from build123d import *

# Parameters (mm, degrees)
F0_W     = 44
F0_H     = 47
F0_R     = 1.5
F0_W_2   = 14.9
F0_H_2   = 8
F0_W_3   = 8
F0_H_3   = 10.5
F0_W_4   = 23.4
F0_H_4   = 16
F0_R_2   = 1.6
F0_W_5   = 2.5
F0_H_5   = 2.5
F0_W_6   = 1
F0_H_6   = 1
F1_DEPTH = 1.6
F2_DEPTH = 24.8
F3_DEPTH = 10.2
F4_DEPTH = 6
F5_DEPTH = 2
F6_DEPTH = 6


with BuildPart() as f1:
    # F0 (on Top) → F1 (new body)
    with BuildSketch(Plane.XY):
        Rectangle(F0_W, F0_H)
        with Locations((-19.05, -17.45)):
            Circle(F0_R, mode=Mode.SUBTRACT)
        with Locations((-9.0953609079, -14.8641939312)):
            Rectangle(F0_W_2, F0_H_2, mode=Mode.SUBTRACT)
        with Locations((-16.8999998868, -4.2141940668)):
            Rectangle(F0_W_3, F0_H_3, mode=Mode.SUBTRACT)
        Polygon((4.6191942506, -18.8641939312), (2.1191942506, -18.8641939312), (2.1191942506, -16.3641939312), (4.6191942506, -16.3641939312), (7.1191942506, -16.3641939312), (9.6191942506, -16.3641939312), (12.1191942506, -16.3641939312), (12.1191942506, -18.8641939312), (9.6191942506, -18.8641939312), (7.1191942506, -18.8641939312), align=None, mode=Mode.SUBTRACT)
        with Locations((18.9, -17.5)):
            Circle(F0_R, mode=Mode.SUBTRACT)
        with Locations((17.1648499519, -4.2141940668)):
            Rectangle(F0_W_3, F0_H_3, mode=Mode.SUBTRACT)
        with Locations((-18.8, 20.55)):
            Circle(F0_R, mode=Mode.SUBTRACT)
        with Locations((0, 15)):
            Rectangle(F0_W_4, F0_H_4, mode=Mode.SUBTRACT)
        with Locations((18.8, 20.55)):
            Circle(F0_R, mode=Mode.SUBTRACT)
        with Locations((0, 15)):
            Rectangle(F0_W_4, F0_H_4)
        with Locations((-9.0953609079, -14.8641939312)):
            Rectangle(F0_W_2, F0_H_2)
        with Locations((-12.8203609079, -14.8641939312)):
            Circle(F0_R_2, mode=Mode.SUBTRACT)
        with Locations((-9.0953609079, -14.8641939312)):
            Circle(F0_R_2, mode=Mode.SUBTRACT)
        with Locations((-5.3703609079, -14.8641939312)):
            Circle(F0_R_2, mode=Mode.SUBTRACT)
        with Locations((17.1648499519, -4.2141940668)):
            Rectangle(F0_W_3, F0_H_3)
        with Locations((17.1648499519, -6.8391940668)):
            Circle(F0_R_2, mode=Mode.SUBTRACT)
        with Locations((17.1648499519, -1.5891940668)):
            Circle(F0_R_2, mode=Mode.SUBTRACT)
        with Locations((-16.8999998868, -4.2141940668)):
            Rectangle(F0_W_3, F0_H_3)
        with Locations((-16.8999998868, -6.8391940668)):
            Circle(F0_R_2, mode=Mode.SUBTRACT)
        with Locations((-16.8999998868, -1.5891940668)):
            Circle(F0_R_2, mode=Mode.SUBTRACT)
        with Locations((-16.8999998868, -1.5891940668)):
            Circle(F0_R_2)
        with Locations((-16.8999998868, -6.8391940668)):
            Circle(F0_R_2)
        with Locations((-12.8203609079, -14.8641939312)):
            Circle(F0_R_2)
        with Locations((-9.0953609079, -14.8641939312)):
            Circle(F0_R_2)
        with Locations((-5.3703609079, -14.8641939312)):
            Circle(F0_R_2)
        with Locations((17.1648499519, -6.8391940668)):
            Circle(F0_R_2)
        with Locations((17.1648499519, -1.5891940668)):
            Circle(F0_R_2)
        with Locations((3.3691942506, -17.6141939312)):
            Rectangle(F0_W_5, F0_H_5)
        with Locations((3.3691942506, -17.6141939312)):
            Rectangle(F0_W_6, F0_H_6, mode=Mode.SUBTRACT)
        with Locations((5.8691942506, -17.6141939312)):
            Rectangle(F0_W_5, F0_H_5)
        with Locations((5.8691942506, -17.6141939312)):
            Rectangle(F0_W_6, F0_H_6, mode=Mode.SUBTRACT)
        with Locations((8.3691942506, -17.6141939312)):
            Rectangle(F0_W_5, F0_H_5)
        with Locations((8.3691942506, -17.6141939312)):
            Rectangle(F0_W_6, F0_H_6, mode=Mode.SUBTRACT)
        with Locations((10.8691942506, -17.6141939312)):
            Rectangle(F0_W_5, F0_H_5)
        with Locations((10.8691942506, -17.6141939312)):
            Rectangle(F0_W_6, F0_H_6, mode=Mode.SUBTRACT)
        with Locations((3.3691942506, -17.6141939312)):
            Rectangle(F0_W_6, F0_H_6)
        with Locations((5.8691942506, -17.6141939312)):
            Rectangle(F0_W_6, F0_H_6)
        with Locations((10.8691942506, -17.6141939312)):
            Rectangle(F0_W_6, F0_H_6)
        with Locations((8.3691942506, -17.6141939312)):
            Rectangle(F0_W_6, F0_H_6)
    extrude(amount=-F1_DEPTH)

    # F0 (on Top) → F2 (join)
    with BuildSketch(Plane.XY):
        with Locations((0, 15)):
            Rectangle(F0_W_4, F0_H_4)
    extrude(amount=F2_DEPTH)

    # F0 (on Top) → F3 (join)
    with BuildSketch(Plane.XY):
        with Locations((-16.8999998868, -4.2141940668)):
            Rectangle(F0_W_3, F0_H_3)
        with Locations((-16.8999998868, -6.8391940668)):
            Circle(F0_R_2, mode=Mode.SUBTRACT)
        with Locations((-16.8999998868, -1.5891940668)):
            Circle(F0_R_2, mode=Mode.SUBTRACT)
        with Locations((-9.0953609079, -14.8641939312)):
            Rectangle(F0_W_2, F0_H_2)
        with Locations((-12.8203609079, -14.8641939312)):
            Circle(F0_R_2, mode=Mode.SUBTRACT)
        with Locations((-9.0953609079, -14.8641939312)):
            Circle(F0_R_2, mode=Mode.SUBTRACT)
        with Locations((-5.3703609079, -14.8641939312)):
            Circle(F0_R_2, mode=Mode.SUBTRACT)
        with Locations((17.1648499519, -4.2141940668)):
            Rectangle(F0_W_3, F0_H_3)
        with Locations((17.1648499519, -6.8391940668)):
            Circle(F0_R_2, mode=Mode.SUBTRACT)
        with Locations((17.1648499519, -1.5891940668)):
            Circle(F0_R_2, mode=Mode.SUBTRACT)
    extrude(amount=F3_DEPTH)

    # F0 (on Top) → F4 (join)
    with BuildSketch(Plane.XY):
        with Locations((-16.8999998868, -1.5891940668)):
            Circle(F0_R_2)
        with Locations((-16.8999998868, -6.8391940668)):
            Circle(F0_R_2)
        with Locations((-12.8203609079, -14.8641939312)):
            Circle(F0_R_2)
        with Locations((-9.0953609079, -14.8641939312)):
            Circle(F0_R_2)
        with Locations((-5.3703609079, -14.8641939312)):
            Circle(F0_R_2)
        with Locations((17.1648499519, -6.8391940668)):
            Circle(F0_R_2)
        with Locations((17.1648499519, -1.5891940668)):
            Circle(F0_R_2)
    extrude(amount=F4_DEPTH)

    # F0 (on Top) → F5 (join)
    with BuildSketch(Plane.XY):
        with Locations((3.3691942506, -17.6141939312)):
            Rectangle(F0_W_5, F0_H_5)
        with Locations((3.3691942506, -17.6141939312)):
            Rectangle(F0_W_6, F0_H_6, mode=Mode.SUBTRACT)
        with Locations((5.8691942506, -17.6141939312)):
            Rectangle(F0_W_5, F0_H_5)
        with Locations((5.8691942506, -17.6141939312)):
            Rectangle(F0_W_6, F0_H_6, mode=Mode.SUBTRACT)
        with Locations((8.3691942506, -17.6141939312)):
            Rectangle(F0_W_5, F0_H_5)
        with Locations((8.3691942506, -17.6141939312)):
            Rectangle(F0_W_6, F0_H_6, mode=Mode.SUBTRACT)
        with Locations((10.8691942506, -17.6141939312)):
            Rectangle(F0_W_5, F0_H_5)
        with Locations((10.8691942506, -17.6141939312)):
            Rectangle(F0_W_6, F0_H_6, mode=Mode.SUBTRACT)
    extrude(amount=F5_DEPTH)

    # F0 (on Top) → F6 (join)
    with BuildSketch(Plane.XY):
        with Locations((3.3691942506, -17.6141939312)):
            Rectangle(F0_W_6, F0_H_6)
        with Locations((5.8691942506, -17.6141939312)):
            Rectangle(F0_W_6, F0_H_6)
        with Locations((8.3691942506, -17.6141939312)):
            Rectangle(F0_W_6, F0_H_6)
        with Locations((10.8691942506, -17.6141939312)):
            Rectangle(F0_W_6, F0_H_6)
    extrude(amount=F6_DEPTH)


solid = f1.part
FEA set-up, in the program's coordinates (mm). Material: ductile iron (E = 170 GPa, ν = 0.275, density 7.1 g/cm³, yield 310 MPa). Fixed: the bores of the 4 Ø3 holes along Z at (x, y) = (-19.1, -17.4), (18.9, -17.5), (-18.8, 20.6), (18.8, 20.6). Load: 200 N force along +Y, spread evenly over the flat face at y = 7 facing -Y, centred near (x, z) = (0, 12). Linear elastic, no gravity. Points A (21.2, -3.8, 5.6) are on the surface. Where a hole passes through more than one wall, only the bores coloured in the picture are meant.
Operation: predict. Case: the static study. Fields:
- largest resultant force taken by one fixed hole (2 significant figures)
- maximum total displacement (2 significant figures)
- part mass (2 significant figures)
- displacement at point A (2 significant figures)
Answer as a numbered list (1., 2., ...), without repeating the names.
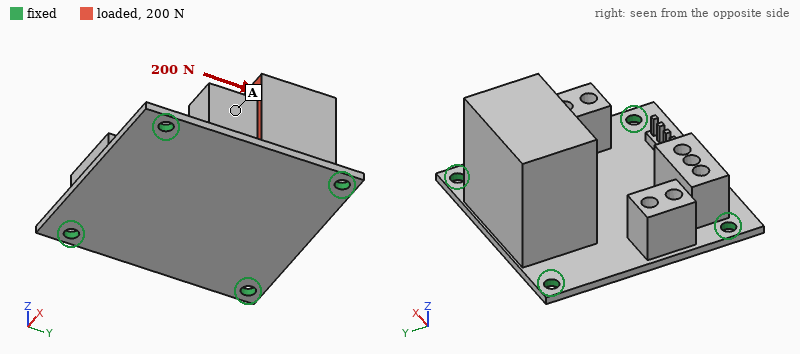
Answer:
1. 77 N
2. 52 µm
3. 110 g
4. 12 µm
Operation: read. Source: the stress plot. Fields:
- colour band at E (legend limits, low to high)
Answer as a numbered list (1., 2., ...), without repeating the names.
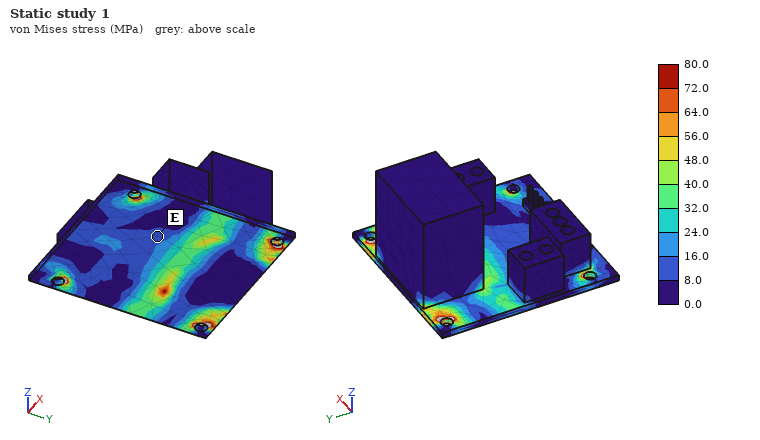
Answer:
1. 8.0 to 16.0 MPa
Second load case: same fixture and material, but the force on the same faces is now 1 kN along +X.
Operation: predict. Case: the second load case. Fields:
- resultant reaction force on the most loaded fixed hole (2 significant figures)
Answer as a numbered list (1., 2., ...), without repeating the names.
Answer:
1. 590 N
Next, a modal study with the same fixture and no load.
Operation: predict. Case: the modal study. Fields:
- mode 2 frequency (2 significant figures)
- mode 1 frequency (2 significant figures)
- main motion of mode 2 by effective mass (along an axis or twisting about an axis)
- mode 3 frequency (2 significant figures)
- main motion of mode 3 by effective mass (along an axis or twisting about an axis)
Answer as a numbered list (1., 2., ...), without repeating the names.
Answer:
1. 3200 Hz
2. 1400 Hz
3. along X
4. 3400 Hz
5. along Z
